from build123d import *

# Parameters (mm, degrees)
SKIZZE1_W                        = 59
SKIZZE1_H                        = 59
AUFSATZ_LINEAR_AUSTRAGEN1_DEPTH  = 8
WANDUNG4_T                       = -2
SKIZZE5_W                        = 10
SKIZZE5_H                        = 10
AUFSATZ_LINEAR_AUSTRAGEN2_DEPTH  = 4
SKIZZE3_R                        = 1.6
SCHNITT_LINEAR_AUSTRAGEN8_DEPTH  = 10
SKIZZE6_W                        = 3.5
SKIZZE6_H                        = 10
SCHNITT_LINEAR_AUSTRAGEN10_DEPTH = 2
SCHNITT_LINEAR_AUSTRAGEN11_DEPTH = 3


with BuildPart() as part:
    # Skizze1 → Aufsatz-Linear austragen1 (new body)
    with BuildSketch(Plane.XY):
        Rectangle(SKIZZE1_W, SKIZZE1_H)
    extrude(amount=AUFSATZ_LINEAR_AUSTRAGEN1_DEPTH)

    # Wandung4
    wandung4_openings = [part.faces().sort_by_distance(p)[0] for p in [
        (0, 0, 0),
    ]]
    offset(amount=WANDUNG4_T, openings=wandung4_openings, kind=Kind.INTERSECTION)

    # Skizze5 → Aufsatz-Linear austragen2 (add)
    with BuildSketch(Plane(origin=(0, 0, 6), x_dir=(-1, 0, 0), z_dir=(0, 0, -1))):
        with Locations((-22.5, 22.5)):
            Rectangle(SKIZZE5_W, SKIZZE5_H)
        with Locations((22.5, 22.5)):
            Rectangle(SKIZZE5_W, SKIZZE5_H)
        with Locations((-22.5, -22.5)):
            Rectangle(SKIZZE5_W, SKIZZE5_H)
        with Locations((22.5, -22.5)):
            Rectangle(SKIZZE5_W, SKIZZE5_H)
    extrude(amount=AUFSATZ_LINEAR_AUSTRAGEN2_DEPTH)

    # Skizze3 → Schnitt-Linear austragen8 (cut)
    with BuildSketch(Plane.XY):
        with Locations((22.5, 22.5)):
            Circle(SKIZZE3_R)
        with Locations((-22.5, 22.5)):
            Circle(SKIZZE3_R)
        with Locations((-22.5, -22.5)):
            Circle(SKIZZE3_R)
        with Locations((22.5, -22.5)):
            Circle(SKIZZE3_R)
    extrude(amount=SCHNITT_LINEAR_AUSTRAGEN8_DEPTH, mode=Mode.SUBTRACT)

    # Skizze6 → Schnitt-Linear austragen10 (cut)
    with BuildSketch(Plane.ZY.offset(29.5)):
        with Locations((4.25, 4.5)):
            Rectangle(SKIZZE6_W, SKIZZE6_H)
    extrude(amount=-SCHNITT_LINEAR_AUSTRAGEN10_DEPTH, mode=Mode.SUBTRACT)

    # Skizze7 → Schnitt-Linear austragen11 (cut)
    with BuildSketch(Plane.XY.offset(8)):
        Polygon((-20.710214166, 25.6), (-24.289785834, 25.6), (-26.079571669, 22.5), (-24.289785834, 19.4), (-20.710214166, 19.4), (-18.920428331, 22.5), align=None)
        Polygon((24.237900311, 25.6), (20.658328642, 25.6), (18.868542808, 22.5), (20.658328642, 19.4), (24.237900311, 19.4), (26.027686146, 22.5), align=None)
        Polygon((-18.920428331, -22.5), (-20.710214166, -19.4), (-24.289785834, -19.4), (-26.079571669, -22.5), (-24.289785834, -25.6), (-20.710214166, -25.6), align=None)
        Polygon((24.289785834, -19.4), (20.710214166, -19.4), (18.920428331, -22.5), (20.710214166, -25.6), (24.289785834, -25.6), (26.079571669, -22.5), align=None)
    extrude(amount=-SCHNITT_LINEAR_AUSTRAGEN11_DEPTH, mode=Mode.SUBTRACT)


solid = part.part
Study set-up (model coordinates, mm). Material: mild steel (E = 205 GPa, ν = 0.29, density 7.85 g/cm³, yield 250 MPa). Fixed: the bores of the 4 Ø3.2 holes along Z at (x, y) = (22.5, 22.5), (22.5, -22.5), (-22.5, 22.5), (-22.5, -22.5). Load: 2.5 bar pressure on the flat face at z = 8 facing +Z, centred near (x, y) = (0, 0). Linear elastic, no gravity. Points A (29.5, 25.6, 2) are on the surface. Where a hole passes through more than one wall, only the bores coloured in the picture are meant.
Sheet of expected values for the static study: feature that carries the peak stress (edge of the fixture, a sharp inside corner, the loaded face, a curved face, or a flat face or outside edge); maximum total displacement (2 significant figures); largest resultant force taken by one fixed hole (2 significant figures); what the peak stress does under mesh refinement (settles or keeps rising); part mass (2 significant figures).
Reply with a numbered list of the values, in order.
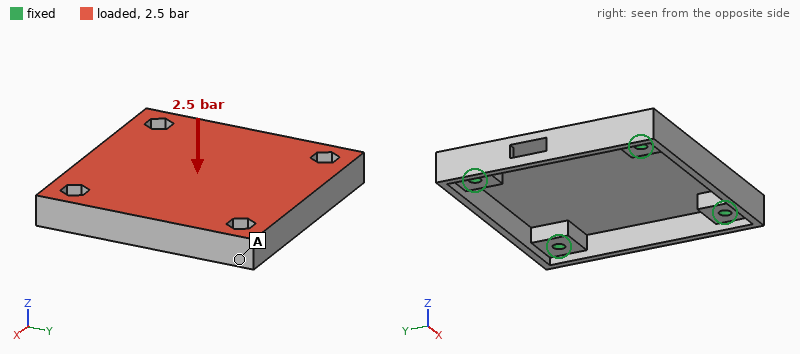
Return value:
1. edge of the fixture
2. 24 µm
3. 310 N
4. keeps rising
5. 84 g
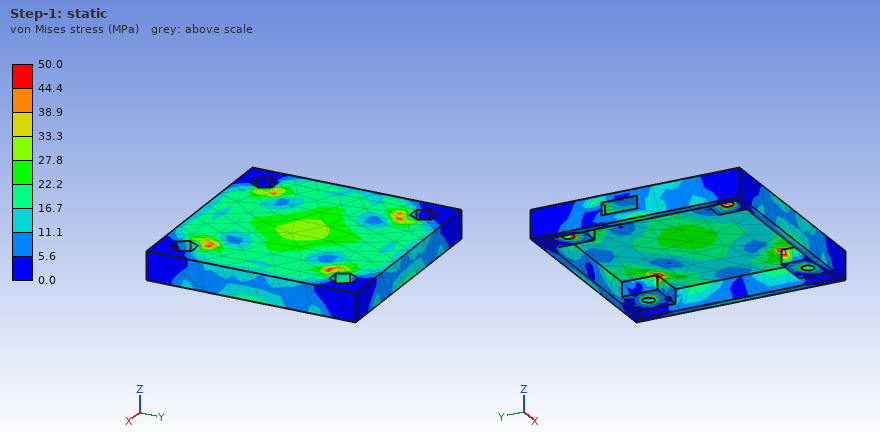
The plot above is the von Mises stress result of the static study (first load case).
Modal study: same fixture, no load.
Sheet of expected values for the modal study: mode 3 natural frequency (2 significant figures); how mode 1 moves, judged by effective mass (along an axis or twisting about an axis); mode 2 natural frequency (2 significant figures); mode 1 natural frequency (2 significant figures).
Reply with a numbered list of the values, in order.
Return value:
1. 9700 Hz
2. along Z
3. 9600 Hz
4. 5100 Hz
